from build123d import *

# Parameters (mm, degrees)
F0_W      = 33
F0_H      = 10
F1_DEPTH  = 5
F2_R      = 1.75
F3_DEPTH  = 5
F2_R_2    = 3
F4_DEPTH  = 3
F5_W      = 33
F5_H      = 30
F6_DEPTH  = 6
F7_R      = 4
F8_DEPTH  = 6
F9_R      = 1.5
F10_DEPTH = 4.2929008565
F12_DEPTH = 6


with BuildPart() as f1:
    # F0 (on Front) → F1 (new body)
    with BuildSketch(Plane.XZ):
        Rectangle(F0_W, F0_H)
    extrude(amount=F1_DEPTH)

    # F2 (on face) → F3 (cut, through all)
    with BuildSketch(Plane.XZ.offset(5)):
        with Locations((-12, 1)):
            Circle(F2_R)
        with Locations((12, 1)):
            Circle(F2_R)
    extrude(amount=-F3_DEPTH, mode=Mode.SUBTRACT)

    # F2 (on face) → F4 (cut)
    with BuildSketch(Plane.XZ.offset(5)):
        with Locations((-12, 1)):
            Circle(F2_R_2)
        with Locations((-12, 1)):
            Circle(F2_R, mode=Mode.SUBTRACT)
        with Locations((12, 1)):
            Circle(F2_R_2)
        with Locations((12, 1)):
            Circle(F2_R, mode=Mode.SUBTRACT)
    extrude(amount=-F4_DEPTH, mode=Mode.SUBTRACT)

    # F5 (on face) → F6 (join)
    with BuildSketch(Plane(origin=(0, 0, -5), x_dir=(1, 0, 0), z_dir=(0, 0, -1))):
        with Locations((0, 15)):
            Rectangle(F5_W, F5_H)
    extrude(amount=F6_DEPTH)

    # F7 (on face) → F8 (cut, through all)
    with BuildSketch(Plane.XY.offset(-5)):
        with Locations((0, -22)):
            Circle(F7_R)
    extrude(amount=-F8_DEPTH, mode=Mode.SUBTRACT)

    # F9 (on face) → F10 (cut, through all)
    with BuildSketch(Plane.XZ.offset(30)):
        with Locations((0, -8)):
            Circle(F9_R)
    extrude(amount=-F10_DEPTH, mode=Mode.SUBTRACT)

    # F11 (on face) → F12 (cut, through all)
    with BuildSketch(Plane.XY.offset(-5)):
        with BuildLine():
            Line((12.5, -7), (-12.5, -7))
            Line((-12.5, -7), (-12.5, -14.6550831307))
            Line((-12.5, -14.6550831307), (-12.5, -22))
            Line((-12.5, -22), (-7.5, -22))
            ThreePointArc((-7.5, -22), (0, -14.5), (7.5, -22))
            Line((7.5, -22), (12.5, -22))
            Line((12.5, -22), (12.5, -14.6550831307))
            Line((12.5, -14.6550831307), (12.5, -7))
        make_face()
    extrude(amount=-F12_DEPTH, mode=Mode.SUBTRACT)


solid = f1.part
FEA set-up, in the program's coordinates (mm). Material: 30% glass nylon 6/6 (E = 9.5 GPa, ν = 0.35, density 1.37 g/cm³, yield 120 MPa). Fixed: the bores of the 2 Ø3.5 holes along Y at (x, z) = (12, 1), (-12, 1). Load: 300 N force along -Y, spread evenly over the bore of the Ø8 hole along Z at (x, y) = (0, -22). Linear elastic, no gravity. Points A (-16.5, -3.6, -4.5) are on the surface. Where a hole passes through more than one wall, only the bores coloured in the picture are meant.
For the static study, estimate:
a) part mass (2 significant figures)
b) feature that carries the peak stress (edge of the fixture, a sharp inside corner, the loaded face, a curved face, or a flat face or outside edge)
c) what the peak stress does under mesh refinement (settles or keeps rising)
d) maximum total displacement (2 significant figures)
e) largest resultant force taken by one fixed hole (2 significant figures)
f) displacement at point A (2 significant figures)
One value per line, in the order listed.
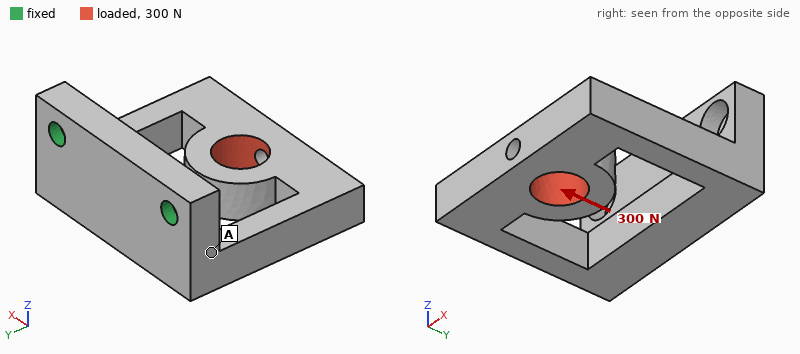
7.3 g
edge of the fixture
keeps rising
0.49 mm
150 N
0.077 mm
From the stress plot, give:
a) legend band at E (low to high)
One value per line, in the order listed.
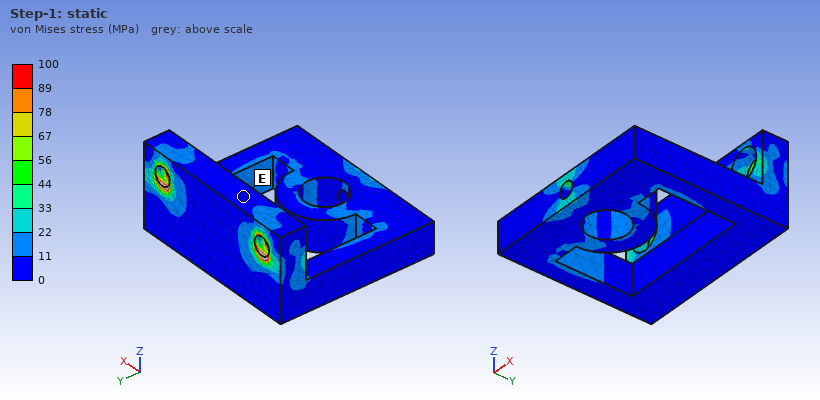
0 to 11 MPa
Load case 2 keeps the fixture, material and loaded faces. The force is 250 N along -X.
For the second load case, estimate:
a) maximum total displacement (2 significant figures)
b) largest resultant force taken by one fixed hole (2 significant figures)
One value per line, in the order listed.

0.47 mm
250 N
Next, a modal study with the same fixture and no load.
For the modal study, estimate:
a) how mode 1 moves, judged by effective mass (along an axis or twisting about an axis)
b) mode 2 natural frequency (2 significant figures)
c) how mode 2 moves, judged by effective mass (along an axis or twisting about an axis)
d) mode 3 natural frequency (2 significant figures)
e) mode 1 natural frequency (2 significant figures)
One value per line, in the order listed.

along Z
2300 Hz
along X
3600 Hz
1100 Hz
